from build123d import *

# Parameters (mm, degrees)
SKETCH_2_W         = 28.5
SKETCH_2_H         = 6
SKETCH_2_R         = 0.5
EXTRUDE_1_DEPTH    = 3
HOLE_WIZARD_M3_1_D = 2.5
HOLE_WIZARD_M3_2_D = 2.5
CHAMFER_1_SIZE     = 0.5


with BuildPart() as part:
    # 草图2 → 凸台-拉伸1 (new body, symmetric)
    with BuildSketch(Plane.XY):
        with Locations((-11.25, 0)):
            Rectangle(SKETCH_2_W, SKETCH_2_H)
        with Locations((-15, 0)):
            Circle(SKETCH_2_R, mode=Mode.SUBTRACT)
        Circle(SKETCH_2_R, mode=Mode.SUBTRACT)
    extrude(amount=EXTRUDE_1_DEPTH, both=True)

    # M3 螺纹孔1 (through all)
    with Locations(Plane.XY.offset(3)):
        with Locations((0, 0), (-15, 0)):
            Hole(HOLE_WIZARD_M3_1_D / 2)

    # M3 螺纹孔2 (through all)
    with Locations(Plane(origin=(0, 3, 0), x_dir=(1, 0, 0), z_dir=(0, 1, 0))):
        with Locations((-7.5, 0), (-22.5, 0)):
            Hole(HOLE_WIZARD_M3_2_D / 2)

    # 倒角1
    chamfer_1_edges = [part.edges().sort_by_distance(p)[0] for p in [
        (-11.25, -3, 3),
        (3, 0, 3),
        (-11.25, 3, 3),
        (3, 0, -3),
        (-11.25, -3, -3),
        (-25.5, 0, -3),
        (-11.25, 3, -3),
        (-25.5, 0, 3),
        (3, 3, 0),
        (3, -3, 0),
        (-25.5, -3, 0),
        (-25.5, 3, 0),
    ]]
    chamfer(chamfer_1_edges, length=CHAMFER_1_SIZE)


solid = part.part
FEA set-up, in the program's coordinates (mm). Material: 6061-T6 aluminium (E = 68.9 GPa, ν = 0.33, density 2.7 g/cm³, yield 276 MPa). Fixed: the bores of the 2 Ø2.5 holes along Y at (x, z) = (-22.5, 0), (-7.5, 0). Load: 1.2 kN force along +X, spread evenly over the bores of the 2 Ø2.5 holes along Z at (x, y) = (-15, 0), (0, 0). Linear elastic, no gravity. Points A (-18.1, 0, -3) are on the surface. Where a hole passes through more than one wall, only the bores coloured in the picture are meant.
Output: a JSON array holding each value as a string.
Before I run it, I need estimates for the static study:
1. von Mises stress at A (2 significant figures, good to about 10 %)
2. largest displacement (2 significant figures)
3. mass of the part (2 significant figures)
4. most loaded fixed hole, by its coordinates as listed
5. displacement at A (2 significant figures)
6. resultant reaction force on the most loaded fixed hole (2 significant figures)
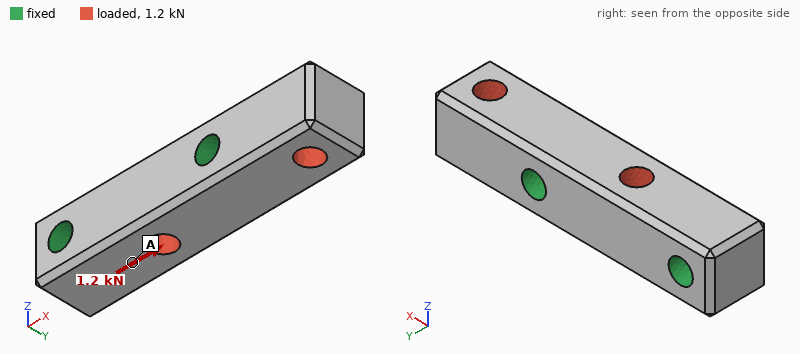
["11 MPa", "3.0 µm", "2.4 g", "(-7.5, 0)", "0.59 µm", "890 N"]
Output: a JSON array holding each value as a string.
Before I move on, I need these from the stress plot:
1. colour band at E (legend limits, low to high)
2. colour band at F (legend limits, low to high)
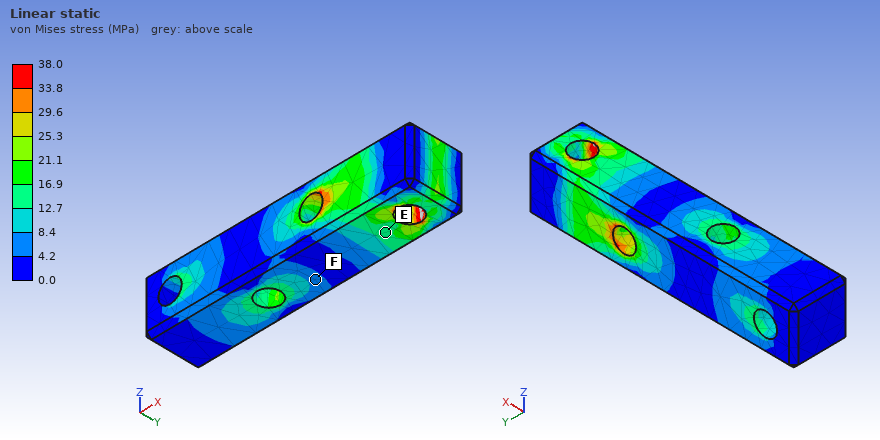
["12.7 to 16.9 MPa", "4.2 to 8.4 MPa"]
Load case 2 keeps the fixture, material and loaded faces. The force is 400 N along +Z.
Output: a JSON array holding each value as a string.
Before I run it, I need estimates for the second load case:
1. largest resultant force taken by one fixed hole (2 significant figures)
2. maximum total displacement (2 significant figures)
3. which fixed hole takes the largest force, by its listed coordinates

["330 N", "10 µm", "(-7.5, 0)"]
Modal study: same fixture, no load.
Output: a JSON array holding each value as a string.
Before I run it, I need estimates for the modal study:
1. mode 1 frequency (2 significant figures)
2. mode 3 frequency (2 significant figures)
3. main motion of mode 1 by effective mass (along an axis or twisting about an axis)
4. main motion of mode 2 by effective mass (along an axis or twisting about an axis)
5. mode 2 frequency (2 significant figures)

["35 kHz", "73 kHz", "along Z", "along Y", "40 kHz"]
